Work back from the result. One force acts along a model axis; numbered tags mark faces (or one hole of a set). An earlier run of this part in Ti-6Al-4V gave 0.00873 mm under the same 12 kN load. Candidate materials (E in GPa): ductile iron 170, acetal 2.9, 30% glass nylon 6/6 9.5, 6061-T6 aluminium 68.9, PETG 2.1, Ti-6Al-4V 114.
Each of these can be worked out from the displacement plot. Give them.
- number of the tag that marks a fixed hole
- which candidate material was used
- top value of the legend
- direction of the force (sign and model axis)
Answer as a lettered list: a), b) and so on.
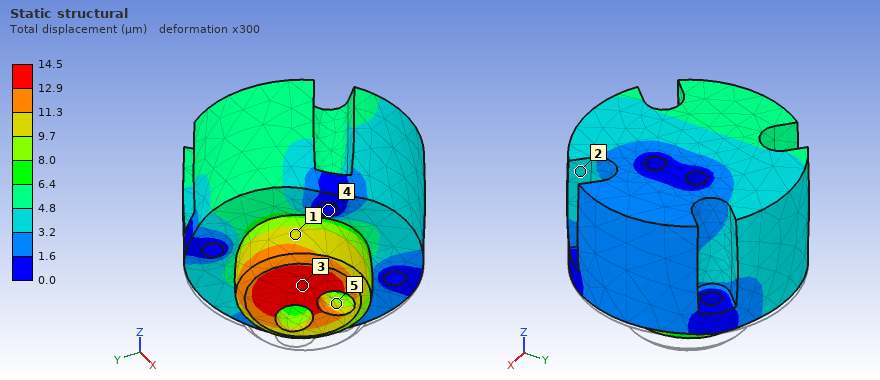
a) 4
b) 6061-T6 aluminium
c) 14.5 µm
d) +Z
